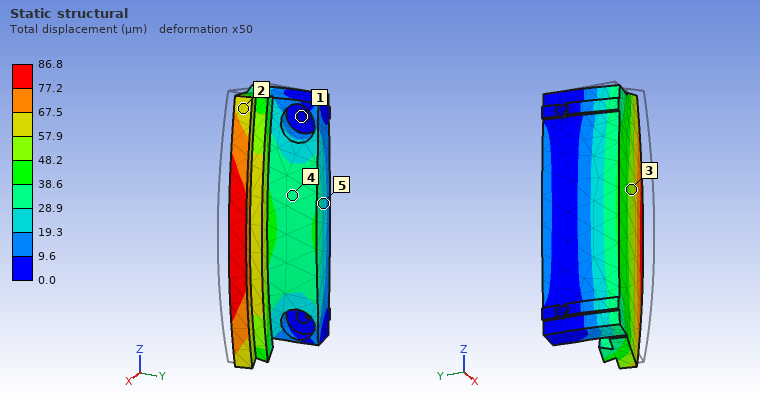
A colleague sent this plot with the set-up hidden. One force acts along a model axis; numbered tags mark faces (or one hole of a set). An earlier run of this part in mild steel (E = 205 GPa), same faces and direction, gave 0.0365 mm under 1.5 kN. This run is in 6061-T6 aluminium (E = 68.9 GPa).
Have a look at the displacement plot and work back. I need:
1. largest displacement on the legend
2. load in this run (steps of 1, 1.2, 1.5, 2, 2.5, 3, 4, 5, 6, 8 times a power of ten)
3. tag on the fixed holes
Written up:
86.8 µm
1.2 kN
1
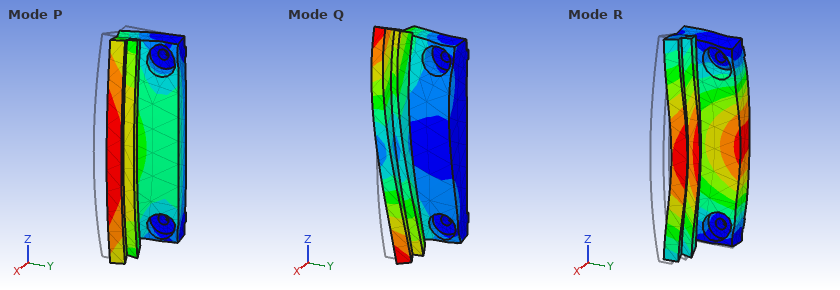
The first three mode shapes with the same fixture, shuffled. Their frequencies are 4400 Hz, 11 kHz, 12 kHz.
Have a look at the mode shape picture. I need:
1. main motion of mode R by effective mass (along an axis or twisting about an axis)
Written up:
along X
